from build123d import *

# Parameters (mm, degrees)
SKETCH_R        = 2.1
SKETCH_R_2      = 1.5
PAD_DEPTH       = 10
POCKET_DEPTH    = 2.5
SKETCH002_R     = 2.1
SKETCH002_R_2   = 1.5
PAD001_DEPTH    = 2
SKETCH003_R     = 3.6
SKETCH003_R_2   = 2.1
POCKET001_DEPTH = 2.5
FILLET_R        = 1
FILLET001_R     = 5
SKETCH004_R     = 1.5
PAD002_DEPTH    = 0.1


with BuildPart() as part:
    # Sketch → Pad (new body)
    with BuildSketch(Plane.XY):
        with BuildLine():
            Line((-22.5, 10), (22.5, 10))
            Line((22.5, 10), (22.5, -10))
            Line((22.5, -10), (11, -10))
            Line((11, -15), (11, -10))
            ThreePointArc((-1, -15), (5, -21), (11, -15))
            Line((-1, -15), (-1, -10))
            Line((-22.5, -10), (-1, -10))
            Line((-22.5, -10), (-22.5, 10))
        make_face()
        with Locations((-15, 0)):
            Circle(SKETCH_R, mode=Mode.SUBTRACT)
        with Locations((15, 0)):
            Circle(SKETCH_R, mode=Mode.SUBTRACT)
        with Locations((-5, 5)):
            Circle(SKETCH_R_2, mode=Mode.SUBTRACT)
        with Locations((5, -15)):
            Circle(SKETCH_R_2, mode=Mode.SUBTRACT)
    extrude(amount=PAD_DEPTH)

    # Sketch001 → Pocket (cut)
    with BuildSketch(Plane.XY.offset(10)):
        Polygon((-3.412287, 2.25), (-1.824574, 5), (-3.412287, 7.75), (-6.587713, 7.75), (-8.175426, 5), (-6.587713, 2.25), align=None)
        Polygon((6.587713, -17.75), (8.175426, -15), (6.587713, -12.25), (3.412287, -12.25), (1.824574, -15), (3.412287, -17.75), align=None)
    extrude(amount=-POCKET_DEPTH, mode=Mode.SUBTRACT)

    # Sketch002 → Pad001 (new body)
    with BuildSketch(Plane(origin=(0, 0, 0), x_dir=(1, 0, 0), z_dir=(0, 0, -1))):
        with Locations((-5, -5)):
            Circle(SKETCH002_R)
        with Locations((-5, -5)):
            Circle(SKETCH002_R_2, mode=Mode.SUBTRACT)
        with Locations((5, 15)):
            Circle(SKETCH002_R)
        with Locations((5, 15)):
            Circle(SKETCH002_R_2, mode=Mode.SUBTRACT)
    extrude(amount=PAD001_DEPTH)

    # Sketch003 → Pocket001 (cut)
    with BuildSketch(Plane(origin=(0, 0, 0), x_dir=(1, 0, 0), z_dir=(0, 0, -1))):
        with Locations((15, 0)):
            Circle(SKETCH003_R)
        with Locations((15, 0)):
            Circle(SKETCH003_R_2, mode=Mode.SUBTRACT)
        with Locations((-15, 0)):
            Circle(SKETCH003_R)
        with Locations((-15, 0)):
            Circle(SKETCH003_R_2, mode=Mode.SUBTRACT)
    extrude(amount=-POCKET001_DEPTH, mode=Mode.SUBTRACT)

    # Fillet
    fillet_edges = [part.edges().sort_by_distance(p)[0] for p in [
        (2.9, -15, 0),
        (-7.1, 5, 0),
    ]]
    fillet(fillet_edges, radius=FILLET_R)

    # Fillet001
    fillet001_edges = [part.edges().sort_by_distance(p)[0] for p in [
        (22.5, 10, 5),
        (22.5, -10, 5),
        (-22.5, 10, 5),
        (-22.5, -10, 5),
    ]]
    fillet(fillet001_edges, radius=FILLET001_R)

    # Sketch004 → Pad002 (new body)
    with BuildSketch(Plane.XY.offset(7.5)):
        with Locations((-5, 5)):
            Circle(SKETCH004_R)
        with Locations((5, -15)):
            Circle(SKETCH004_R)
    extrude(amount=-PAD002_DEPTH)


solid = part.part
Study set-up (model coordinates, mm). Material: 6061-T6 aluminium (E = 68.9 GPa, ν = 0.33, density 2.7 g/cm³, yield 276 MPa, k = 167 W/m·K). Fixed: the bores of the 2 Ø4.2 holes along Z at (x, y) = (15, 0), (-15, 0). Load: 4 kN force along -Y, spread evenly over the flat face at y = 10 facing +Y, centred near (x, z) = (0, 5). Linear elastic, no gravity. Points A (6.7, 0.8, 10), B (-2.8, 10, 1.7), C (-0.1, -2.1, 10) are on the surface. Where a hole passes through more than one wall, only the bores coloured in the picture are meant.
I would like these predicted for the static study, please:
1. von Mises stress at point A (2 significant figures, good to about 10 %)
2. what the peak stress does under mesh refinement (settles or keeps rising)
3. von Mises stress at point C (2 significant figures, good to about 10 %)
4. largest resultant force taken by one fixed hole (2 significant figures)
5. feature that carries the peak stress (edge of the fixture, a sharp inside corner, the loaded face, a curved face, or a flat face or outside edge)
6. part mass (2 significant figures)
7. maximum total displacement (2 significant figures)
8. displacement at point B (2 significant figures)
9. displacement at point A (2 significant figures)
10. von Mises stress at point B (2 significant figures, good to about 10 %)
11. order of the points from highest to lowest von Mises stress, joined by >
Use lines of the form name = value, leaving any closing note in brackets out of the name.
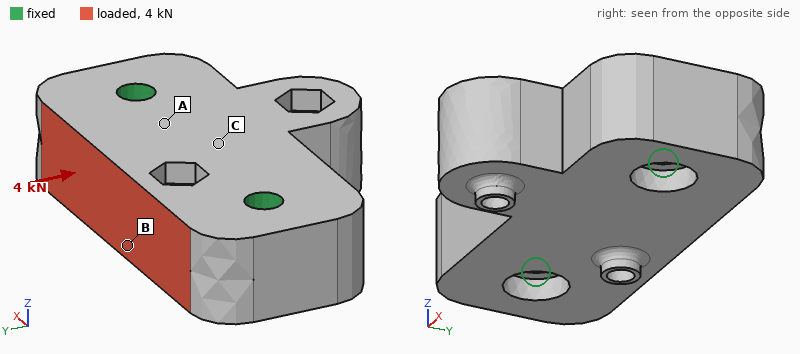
von Mises stress at point A = 9.0 MPa
what the peak stress does under mesh refinement = keeps rising
von Mises stress at point C = 5.3 MPa
largest resultant force taken by one fixed hole = 2.0 kN
feature that carries the peak stress = edge of the fixture
part mass = 25 g
maximum total displacement = 7.4 µm
displacement at point B = 6.9 µm
displacement at point A = 3.0 µm
von Mises stress at point B = 17 MPa
order of the points from highest to lowest von Mises stress, joined by > = B > A > C
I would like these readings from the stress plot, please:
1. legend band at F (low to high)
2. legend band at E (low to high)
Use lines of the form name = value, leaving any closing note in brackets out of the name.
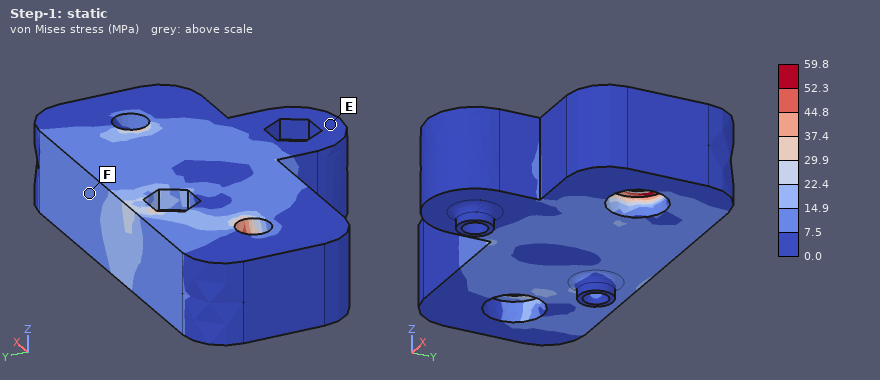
legend band at F = 7.5 to 14.9 MPa
legend band at E = 0.0 to 7.5 MPa
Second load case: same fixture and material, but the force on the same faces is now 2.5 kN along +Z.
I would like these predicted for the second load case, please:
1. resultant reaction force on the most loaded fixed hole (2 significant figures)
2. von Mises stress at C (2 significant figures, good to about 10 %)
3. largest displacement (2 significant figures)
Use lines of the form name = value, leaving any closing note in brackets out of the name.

resultant reaction force on the most loaded fixed hole = 1.3 kN
von Mises stress at C = 17 MPa
largest displacement = 23 µm
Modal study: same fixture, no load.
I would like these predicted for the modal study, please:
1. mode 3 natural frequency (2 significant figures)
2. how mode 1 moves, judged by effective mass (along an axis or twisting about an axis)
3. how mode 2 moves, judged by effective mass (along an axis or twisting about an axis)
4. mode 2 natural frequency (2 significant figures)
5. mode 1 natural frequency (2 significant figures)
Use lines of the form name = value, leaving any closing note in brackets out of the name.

mode 3 natural frequency = 30 kHz
how mode 1 moves, judged by effective mass = along Z
how mode 2 moves, judged by effective mass = along Z
mode 2 natural frequency = 28 kHz
mode 1 natural frequency = 16 kHz
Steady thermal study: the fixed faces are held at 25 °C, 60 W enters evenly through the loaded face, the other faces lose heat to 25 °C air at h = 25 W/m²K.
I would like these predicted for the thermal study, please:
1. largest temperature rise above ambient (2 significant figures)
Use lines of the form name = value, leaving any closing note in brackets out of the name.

largest temperature rise above ambient = 16 K
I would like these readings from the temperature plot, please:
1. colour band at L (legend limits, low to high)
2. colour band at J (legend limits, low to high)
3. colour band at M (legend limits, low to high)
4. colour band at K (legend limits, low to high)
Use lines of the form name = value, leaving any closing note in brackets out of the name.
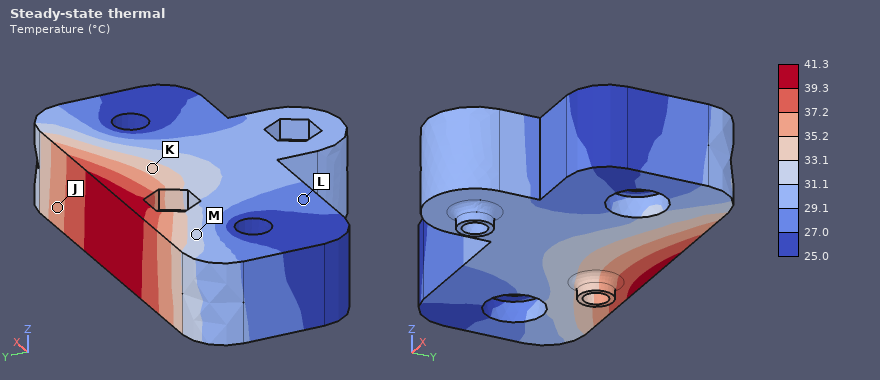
colour band at L = 27.0 to 29.1 °C
colour band at J = 35.2 to 37.2 °C
colour band at M = 31.1 to 33.1 °C
colour band at K = 33.1 to 35.2 °C
